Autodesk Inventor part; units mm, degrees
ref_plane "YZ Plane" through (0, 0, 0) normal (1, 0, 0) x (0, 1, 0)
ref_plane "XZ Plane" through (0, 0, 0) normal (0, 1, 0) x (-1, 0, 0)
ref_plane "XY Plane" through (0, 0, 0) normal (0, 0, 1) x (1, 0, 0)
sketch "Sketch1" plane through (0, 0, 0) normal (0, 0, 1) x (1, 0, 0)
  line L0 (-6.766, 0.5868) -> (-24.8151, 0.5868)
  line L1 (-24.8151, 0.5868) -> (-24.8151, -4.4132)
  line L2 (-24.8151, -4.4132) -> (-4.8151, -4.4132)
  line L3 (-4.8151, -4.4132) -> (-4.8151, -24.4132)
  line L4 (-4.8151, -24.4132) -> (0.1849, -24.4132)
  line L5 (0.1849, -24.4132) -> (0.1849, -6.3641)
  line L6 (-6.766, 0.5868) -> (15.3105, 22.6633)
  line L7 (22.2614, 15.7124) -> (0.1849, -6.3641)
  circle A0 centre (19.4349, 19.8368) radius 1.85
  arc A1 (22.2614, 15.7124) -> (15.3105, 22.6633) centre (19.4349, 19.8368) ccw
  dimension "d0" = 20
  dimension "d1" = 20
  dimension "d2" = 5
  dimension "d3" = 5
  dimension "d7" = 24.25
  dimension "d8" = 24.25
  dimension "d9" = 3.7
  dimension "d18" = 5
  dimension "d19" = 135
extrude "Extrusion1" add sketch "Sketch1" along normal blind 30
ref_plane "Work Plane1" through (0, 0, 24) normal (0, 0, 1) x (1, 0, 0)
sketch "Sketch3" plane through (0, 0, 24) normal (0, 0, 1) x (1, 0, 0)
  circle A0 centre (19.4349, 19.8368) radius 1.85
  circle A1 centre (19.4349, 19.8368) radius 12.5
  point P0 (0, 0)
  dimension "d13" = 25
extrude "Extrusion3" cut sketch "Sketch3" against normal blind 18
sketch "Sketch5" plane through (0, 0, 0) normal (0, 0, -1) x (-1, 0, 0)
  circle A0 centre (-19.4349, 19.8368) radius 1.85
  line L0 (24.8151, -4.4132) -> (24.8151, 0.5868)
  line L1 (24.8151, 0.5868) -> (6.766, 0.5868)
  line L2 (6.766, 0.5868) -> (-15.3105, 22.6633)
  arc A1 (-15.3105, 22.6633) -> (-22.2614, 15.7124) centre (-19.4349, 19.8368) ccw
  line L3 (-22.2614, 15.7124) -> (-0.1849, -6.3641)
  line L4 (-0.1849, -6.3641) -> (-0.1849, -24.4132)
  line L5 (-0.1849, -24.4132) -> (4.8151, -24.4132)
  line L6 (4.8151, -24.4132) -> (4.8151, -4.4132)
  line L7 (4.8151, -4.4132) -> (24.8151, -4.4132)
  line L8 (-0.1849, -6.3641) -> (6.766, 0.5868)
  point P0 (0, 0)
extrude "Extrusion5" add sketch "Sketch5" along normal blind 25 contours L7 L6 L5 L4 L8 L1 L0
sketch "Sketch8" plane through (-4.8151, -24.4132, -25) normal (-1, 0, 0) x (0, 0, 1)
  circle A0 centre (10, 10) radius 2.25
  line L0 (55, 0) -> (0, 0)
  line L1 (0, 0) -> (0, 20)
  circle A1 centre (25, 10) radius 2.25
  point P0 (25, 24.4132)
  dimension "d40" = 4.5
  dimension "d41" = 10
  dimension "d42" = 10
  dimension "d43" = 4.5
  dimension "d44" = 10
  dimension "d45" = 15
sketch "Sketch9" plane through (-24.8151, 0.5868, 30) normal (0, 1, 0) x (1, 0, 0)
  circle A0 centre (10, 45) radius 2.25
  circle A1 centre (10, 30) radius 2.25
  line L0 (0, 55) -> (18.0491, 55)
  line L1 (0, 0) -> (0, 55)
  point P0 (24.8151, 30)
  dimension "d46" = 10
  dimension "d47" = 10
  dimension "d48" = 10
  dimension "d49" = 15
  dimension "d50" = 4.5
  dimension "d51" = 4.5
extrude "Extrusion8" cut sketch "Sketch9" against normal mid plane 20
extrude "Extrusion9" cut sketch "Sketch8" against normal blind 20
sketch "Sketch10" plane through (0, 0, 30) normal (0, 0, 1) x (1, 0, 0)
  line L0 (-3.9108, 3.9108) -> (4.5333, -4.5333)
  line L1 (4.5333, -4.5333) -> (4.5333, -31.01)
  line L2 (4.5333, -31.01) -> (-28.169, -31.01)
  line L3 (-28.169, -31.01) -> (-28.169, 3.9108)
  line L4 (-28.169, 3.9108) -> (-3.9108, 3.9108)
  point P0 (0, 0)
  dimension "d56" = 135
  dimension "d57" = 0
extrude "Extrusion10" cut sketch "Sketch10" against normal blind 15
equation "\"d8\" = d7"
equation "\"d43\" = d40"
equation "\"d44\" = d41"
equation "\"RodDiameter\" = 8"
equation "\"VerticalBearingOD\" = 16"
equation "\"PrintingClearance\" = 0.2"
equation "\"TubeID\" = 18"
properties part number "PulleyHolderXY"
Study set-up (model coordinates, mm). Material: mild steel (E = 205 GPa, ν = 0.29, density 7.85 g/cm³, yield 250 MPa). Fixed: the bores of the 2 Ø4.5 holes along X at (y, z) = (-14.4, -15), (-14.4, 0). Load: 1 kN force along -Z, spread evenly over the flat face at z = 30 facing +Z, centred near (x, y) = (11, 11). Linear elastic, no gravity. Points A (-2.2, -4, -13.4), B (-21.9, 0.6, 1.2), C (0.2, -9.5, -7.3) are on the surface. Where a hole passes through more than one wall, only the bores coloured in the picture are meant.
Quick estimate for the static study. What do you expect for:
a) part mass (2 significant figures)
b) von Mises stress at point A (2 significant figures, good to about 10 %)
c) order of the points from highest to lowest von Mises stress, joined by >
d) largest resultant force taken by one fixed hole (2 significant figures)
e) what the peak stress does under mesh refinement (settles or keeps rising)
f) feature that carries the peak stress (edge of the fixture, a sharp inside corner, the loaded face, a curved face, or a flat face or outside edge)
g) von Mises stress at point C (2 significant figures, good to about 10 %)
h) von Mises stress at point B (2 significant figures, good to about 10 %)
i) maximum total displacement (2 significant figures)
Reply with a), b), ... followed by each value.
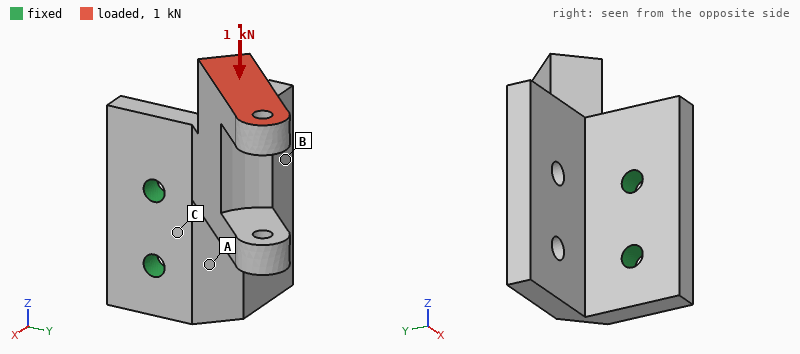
a) 120 g
b) 35 MPa
c) C > A > B
d) 1.3 kN
e) keeps rising
f) edge of the fixture
g) 56 MPa
h) 13 MPa
i) 0.10 mm
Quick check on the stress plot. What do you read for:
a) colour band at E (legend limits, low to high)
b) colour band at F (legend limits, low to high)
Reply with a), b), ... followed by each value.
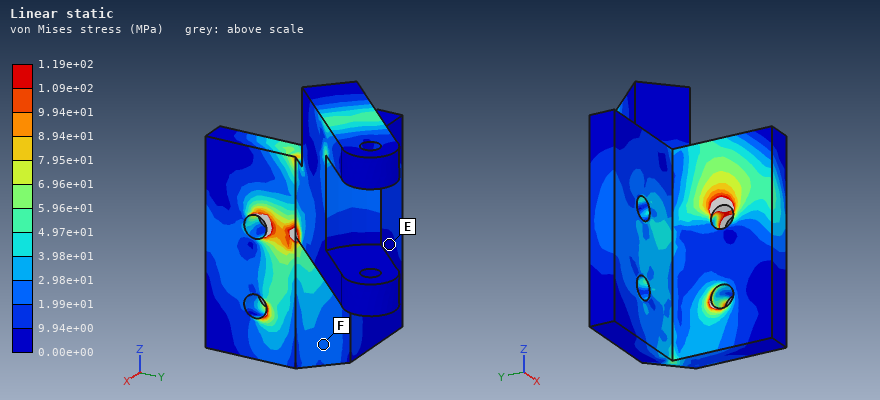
a) 0.00e+00 to 9.94e+00 MPa
b) 1.99e+01 to 2.98e+01 MPa
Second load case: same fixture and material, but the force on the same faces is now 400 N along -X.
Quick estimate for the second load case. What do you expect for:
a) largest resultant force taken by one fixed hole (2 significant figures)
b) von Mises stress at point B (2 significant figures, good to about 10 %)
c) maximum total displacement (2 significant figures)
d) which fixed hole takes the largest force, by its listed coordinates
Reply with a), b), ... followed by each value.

a) 830 N
b) 16 MPa
c) 0.14 mm
d) (-14.4, 0)
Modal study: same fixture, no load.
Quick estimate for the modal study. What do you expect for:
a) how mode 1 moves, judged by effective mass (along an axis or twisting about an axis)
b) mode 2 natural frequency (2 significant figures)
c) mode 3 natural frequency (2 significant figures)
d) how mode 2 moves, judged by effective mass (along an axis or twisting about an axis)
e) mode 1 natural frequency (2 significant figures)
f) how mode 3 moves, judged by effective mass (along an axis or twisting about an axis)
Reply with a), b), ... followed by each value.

a) along X
b) 3300 Hz
c) 5100 Hz
d) along Z
e) 1700 Hz
f) along Y
